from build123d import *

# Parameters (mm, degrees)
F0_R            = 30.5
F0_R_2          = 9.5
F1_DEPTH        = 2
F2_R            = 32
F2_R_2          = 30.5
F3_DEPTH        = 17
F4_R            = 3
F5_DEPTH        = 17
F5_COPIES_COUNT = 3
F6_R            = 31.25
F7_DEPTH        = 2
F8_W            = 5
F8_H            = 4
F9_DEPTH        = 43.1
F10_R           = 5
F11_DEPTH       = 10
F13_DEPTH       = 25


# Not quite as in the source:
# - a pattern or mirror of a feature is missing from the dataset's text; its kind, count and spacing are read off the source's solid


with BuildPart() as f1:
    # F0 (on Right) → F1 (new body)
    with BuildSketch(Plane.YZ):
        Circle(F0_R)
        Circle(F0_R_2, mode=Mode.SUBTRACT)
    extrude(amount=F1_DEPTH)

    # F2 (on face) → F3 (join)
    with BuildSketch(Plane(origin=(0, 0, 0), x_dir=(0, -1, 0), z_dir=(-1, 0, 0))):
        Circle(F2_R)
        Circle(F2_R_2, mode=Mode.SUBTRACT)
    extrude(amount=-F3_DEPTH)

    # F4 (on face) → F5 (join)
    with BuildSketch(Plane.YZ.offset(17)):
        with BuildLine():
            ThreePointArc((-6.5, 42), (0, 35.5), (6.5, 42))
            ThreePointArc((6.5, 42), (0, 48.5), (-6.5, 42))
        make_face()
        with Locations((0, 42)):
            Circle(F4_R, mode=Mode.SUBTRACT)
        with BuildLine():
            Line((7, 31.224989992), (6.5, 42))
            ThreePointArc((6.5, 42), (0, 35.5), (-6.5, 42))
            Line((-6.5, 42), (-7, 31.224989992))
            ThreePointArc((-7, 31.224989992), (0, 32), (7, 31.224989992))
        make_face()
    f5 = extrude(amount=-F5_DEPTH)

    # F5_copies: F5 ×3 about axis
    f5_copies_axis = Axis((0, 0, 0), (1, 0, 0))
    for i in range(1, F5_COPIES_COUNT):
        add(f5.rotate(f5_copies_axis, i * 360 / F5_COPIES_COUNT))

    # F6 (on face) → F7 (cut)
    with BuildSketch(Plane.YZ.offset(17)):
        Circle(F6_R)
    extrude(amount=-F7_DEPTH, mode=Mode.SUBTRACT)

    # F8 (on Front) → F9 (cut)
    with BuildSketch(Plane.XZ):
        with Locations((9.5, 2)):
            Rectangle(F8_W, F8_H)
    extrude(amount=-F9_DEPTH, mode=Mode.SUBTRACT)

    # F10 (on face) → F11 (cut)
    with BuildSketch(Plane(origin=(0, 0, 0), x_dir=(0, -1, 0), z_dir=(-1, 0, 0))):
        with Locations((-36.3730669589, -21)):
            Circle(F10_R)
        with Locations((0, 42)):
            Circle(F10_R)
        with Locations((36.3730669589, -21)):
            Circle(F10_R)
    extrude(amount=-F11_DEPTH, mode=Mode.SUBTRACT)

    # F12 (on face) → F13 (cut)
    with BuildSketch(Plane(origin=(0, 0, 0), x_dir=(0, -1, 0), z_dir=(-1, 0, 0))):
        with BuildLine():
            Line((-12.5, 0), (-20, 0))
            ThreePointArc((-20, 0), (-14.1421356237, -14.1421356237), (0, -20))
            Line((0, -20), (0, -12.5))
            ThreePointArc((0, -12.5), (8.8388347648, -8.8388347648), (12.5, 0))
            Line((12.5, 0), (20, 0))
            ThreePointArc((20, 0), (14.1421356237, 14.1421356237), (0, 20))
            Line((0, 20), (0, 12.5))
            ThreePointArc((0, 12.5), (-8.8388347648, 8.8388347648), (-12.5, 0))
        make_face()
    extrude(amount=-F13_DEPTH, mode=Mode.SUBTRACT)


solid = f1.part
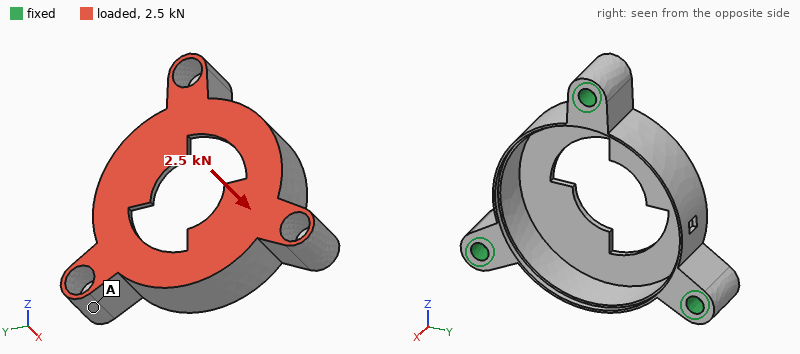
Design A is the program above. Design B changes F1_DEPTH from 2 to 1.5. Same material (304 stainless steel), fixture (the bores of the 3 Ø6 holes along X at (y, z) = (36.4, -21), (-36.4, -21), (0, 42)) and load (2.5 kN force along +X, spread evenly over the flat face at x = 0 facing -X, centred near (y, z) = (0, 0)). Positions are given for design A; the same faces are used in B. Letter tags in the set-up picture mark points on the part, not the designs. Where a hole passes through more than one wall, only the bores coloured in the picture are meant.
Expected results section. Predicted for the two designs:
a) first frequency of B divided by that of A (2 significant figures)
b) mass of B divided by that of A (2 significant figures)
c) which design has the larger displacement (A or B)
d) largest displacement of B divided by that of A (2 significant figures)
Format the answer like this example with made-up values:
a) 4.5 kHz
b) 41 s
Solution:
a) 0.85
b) 0.94
c) B
d) 1.9
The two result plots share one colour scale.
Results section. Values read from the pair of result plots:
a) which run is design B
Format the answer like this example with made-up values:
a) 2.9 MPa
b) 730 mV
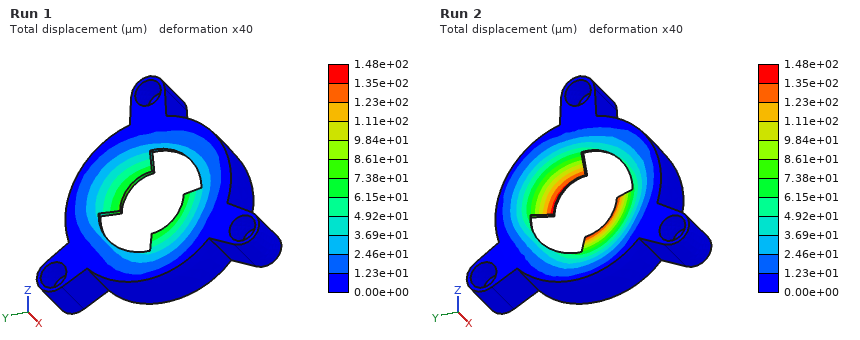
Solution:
a) Run 2
